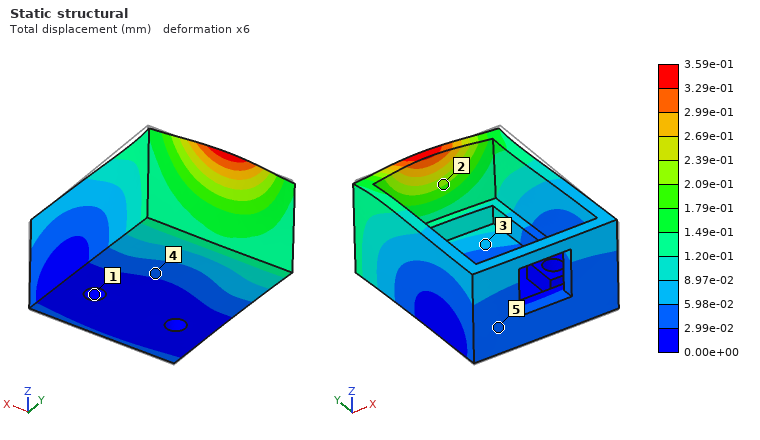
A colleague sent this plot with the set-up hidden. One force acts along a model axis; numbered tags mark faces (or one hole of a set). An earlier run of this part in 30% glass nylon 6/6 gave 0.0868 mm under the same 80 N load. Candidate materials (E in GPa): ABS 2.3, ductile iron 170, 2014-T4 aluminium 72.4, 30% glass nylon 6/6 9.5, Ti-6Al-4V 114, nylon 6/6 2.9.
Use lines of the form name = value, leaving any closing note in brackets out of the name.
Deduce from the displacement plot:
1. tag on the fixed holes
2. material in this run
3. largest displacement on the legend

tag on the fixed holes = 1
material in this run = ABS
largest displacement on the legend = 3.59e-01 mm
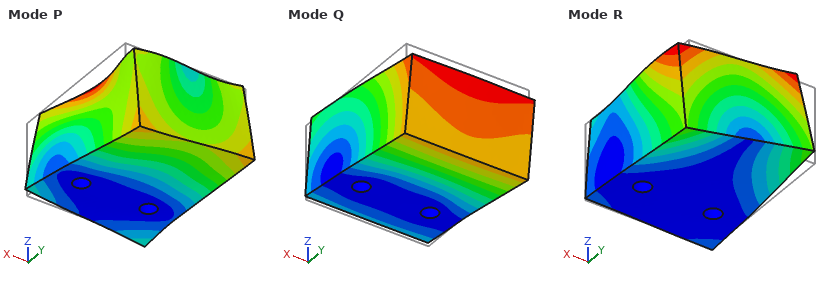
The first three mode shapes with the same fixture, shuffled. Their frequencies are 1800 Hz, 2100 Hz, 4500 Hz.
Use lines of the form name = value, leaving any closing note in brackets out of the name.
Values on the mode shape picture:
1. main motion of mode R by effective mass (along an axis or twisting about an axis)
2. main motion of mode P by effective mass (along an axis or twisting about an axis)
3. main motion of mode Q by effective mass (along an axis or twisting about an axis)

main motion of mode R by effective mass = along X
main motion of mode P by effective mass = along X
main motion of mode Q by effective mass = along Z
